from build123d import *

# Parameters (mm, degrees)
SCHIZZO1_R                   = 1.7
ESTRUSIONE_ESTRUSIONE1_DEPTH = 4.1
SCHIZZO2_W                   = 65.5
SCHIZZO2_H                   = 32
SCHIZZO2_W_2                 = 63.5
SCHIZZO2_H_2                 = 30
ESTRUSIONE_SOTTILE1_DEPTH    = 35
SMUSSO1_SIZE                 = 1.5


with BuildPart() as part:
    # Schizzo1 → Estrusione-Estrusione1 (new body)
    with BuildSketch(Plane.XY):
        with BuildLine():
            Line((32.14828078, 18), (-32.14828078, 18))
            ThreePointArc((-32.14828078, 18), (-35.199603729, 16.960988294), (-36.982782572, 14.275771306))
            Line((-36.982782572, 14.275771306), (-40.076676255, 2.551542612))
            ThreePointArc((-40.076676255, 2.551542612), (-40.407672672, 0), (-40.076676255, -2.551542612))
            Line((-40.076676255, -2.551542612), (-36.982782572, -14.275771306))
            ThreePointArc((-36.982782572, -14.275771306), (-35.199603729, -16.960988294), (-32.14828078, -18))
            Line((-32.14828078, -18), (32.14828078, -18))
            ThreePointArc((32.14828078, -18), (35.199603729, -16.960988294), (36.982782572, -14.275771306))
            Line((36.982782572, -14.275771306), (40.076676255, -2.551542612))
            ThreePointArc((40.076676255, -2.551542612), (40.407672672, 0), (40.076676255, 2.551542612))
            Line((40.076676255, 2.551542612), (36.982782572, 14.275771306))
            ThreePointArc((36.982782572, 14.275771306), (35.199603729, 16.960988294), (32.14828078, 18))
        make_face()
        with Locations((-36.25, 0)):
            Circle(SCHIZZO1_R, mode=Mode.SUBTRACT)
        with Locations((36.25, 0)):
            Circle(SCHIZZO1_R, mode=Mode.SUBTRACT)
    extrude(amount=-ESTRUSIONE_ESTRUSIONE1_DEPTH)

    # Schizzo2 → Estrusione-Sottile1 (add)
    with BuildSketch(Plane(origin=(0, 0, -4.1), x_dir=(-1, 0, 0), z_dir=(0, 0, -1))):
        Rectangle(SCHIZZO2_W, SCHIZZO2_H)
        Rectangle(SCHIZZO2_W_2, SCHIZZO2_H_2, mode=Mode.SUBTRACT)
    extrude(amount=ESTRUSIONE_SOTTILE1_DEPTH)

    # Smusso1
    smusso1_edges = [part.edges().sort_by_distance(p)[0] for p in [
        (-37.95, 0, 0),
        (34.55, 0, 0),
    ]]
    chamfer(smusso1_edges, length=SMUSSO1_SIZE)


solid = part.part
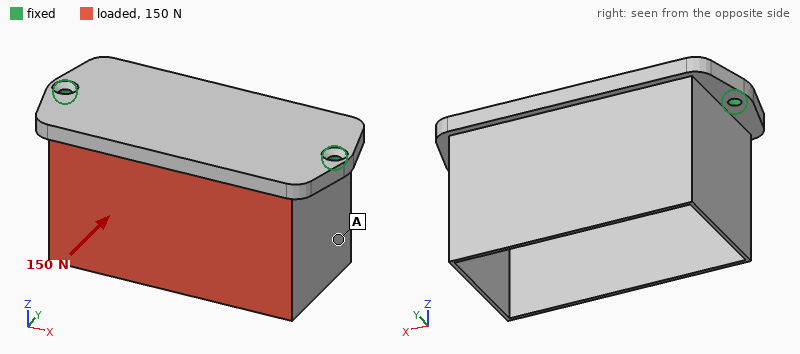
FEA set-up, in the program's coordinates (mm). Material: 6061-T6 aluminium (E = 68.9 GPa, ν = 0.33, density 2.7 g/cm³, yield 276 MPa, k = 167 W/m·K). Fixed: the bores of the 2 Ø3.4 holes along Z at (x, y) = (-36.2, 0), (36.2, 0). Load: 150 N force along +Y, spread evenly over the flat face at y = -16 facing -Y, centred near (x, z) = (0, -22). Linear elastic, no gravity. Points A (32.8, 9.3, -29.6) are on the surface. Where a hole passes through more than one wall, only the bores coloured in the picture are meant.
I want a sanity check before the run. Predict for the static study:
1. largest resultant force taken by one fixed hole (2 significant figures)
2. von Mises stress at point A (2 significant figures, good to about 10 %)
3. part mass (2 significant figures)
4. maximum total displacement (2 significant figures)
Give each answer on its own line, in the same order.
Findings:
75 N
8.9 MPa
48 g
0.58 mm
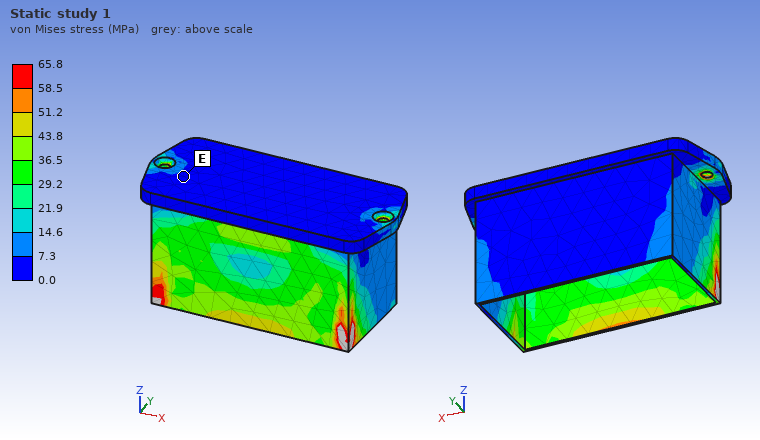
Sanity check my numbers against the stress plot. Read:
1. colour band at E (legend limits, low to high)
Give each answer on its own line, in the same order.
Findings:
0.0 to 7.3 MPa
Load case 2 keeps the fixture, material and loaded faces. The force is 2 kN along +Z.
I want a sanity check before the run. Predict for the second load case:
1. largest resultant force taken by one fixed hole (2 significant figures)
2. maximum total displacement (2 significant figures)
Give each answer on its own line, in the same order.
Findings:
1.0 kN
0.84 mm
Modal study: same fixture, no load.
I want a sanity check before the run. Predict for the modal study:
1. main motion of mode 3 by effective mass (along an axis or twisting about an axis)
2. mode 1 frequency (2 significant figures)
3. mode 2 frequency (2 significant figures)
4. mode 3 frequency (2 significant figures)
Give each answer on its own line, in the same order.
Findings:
twisting about X
1400 Hz
1400 Hz
2600 Hz
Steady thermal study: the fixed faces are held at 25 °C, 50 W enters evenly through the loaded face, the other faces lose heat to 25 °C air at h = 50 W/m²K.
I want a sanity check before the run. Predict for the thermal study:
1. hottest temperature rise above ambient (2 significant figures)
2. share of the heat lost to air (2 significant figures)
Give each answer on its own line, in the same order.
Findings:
69 K
35 %
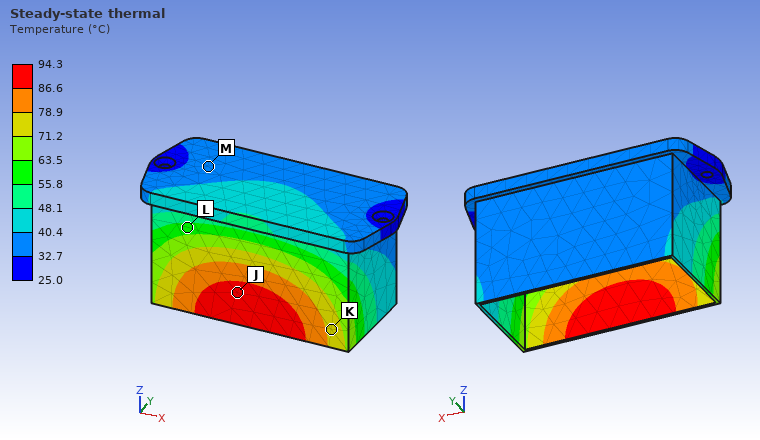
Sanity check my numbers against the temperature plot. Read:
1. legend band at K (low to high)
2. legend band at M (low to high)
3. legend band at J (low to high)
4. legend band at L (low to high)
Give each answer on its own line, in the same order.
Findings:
71.2 to 78.9 °C
32.7 to 40.4 °C
86.6 to 94.3 °C
55.8 to 63.5 °C
